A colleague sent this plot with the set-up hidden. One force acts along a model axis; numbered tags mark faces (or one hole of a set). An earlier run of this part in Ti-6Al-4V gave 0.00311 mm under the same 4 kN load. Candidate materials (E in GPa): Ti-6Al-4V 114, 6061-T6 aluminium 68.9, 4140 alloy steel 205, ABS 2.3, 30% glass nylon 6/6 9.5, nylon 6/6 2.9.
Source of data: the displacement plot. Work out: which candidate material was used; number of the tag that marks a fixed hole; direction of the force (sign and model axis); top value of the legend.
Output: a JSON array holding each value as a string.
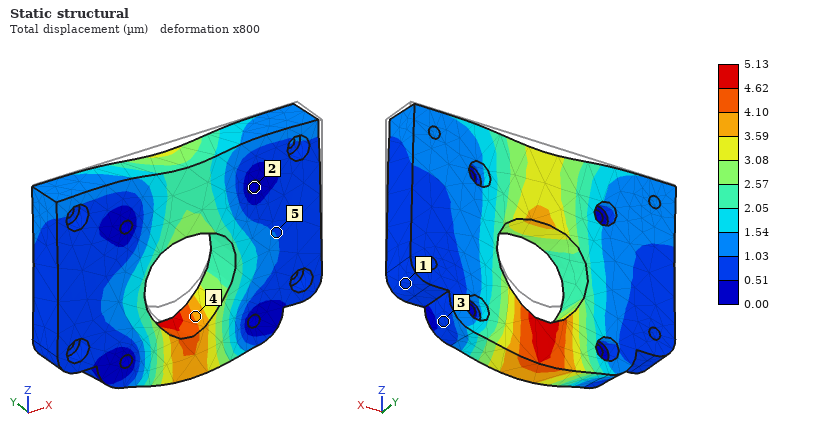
["6061-T6 aluminium", "2", "-Z", "5.13 µm"]
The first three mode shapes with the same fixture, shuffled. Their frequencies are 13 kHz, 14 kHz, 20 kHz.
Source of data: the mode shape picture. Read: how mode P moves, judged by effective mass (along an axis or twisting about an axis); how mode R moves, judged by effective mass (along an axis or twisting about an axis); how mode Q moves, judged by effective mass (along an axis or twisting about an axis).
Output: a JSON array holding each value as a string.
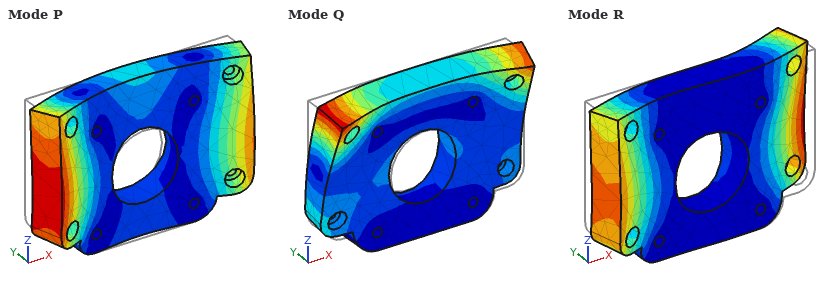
["along Y", "twisting about Z", "twisting about X"]
